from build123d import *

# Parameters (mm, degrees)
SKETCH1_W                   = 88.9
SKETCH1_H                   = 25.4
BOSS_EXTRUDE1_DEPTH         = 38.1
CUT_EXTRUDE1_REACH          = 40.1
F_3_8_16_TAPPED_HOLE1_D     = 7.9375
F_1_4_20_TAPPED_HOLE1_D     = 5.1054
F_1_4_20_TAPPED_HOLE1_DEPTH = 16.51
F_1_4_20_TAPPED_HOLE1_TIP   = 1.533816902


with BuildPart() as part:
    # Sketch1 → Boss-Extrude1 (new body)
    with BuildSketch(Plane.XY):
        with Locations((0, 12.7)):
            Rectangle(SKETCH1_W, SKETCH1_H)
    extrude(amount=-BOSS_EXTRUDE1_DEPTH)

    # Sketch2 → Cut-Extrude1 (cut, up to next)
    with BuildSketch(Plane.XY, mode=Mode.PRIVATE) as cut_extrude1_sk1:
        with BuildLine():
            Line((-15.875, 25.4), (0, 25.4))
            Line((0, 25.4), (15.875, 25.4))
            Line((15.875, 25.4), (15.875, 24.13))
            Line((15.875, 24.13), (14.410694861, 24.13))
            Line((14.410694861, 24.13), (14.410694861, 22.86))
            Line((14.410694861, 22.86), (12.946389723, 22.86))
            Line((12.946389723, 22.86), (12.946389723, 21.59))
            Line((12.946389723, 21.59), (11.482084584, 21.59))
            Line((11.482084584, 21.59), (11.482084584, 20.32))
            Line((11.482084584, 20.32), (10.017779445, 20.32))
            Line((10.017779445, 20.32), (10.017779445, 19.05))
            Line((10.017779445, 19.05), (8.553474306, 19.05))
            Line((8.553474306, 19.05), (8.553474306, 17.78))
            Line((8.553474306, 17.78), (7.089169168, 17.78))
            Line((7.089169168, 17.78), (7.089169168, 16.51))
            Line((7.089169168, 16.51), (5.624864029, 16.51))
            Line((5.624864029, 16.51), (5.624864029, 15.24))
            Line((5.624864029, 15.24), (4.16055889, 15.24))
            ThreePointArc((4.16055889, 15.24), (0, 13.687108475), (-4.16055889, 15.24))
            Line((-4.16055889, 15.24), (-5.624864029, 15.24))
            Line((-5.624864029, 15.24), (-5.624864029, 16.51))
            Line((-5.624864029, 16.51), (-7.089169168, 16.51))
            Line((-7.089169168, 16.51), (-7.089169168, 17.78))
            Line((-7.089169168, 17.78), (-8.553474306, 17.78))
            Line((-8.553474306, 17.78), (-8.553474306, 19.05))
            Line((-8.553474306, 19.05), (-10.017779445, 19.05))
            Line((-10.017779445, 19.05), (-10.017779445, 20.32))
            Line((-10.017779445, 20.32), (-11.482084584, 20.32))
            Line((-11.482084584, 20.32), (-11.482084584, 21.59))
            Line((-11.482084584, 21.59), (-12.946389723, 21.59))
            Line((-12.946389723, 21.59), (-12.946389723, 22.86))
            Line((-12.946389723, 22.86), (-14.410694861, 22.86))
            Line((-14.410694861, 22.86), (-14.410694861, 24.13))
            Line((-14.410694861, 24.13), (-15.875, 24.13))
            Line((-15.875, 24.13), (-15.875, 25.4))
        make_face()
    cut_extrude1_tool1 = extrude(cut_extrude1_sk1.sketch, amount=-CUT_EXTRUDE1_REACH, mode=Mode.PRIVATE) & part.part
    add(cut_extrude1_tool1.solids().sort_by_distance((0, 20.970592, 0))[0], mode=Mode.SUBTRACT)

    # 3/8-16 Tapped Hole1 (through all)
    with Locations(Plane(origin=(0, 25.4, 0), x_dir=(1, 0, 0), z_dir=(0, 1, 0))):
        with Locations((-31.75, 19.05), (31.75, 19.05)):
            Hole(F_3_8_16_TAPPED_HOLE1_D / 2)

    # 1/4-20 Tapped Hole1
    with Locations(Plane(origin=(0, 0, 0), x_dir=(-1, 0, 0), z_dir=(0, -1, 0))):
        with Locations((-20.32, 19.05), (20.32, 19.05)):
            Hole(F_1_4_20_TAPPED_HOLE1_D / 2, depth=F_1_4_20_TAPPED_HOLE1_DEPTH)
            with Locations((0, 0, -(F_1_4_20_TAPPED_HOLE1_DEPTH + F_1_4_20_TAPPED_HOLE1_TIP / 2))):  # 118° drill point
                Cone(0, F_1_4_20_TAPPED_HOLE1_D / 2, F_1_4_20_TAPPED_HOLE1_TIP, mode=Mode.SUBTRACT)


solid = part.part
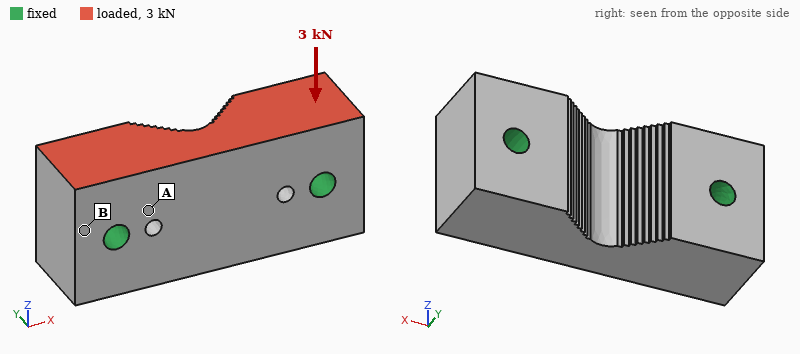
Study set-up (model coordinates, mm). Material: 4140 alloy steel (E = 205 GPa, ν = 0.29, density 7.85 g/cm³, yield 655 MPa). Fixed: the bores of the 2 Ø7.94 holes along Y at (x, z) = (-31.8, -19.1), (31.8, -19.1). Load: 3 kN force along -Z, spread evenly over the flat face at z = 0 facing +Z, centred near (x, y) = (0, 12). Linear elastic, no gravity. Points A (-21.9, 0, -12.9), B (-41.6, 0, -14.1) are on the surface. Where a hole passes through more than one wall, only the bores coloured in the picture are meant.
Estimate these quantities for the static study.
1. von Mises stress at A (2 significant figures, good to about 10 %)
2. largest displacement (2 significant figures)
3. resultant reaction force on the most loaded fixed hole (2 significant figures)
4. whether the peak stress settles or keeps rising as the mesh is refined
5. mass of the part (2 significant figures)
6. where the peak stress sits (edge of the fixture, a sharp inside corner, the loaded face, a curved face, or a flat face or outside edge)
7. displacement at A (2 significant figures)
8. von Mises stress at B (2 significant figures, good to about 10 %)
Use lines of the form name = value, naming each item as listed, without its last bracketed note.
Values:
von Mises stress at A = 3.2 MPa
largest displacement = 0.63 µm
resultant reaction force on the most loaded fixed hole = 1.5 kN
whether the peak stress settles or keeps rising as the mesh is refined = keeps rising
mass of the part = 580 g
where the peak stress sits = edge of the fixture
displacement at A = 0.25 µm
von Mises stress at B = 0.86 MPa
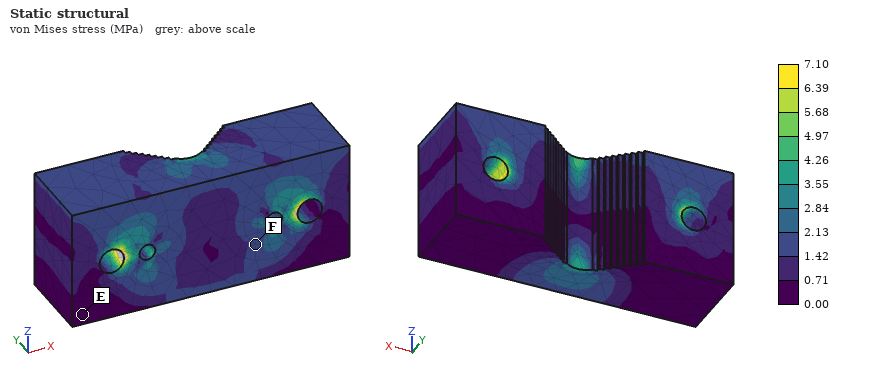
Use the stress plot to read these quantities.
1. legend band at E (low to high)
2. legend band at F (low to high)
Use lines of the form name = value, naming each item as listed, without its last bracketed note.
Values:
legend band at E = 0.00 to 0.71 MPa
legend band at F = 1.42 to 2.13 MPa
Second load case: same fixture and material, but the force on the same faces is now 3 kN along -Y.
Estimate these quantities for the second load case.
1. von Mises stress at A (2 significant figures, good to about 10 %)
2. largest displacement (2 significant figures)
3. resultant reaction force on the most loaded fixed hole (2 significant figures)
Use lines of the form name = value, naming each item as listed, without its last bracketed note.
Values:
von Mises stress at A = 5.3 MPa
largest displacement = 1.9 µm
resultant reaction force on the most loaded fixed hole = 1.5 kN
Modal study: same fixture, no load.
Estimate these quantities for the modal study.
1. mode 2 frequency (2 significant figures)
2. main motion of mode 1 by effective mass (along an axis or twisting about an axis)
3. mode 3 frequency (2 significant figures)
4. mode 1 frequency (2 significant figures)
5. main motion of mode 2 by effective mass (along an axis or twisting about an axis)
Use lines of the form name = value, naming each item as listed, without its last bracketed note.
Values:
mode 2 frequency = 17 kHz
main motion of mode 1 by effective mass = along Z
mode 3 frequency = 22 kHz
mode 1 frequency = 16 kHz
main motion of mode 2 by effective mass = along Y
